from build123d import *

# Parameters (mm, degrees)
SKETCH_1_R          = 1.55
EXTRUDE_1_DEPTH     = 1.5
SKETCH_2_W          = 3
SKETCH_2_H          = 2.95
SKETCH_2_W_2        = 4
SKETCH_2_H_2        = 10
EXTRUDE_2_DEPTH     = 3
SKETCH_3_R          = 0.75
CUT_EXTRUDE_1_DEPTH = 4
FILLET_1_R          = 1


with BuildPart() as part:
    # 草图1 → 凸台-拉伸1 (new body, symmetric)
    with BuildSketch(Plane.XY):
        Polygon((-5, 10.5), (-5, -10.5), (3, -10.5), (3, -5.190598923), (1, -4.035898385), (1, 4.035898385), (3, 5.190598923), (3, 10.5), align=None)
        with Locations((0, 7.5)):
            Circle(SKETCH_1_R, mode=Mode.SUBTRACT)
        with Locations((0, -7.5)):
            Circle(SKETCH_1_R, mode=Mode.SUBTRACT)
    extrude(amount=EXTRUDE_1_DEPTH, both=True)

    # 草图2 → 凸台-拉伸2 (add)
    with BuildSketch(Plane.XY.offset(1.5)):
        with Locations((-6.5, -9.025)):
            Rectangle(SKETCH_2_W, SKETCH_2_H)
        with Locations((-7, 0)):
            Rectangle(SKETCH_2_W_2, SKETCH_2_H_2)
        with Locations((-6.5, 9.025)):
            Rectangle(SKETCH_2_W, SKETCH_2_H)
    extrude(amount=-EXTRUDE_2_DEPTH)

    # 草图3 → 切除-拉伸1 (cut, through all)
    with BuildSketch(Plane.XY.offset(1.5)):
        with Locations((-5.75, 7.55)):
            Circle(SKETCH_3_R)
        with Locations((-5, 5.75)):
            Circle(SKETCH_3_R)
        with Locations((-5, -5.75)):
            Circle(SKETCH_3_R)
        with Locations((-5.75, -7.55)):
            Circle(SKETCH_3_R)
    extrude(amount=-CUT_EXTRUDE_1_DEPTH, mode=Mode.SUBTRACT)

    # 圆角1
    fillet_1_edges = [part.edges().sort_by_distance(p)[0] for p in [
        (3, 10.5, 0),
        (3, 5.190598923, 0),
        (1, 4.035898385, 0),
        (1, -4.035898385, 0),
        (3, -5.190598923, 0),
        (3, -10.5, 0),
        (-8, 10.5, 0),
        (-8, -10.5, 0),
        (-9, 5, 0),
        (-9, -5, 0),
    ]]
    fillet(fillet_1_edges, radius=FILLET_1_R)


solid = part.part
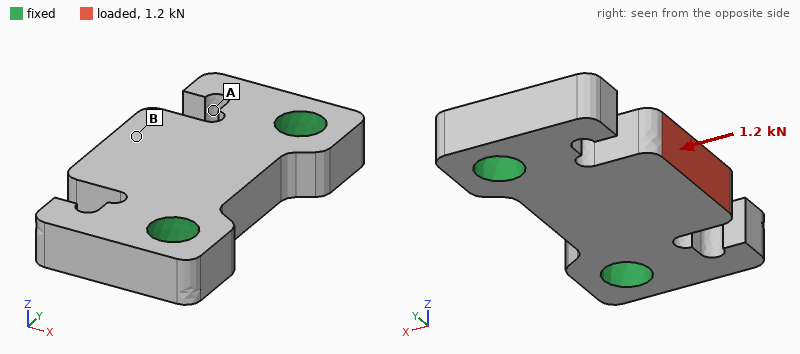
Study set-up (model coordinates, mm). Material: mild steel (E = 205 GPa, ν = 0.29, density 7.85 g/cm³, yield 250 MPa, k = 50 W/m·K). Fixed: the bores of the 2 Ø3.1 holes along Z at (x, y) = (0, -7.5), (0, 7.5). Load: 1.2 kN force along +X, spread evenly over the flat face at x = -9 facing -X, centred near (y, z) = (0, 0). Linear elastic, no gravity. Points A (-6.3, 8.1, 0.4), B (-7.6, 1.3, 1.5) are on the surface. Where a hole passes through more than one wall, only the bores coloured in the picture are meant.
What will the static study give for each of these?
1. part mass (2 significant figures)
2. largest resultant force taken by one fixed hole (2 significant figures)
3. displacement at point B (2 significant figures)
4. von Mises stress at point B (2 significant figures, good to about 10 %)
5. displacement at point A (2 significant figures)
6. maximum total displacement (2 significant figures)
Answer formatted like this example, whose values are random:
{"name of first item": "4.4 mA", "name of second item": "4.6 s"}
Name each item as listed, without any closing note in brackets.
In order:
{"part mass": "4.4 g", "largest resultant force taken by one fixed hole": "690 N", "displacement at point B": "2.6 µm", "von Mises stress at point B": "43 MPa", "displacement at point A": "0.59 µm", "maximum total displacement": "3.0 µm"}
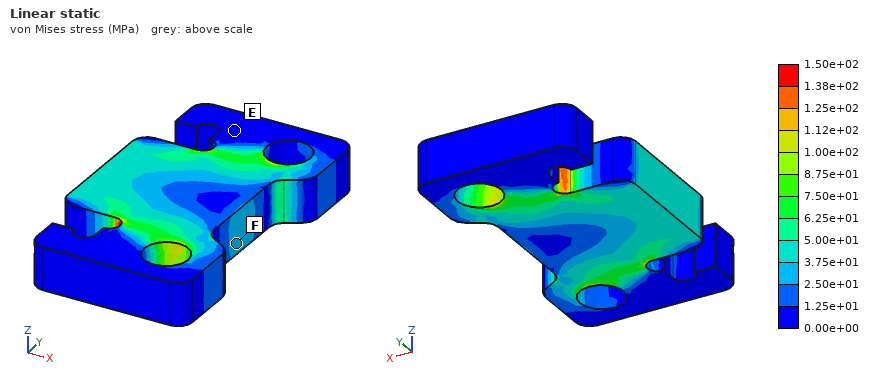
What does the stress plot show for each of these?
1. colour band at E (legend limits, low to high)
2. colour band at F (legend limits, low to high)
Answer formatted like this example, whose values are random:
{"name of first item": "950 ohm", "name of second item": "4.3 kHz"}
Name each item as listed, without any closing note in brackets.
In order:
{"colour band at E": "0.00e+00 to 1.25e+01 MPa", "colour band at F": "2.50e+01 to 3.75e+01 MPa"}
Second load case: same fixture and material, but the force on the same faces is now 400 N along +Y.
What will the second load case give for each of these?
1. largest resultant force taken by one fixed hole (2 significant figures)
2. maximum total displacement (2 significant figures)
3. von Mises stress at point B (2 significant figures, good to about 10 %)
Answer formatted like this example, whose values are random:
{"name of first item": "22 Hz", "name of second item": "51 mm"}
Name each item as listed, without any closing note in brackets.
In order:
{"largest resultant force taken by one fixed hole": "320 N", "maximum total displacement": "2.3 µm", "von Mises stress at point B": "32 MPa"}
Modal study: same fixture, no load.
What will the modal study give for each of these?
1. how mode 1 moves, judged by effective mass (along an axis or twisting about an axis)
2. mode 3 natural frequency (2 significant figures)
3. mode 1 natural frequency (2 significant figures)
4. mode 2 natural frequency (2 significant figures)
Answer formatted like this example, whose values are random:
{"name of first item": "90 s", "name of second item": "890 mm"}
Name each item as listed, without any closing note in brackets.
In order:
{"how mode 1 moves, judged by effective mass": "along Z", "mode 3 natural frequency": "56 kHz", "mode 1 natural frequency": "27 kHz", "mode 2 natural frequency": "55 kHz"}
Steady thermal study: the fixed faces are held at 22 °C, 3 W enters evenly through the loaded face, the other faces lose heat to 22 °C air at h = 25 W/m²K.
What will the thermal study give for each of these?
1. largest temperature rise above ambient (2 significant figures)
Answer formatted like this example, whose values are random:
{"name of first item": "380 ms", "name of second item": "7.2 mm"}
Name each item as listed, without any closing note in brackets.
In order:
{"largest temperature rise above ambient": "19 K"}
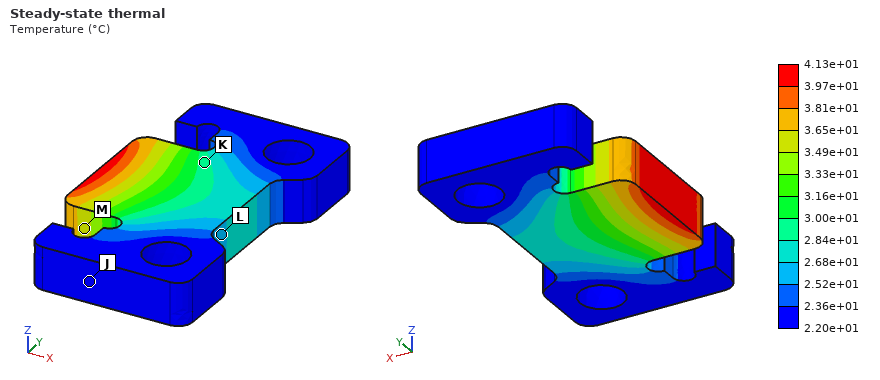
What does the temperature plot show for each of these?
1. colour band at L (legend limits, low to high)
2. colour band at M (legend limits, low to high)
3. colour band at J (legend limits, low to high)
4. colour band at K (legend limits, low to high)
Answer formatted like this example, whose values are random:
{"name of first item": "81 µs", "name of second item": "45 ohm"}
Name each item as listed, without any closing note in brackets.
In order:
{"colour band at L": "2.52e+01 to 2.68e+01 °C", "colour band at M": "3.49e+01 to 3.65e+01 °C", "colour band at J": "2.20e+01 to 2.36e+01 °C", "colour band at K": "2.84e+01 to 3.00e+01 °C"}
